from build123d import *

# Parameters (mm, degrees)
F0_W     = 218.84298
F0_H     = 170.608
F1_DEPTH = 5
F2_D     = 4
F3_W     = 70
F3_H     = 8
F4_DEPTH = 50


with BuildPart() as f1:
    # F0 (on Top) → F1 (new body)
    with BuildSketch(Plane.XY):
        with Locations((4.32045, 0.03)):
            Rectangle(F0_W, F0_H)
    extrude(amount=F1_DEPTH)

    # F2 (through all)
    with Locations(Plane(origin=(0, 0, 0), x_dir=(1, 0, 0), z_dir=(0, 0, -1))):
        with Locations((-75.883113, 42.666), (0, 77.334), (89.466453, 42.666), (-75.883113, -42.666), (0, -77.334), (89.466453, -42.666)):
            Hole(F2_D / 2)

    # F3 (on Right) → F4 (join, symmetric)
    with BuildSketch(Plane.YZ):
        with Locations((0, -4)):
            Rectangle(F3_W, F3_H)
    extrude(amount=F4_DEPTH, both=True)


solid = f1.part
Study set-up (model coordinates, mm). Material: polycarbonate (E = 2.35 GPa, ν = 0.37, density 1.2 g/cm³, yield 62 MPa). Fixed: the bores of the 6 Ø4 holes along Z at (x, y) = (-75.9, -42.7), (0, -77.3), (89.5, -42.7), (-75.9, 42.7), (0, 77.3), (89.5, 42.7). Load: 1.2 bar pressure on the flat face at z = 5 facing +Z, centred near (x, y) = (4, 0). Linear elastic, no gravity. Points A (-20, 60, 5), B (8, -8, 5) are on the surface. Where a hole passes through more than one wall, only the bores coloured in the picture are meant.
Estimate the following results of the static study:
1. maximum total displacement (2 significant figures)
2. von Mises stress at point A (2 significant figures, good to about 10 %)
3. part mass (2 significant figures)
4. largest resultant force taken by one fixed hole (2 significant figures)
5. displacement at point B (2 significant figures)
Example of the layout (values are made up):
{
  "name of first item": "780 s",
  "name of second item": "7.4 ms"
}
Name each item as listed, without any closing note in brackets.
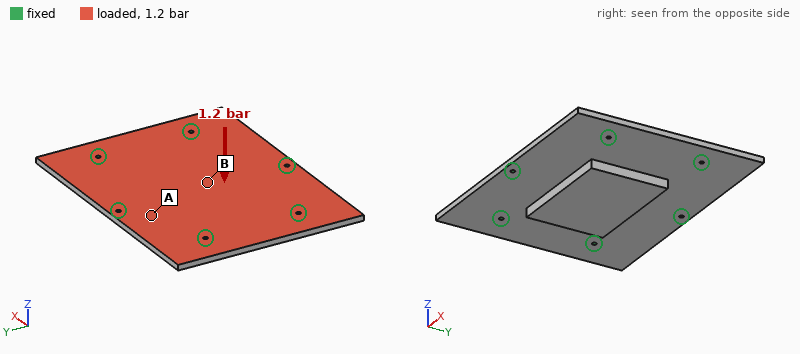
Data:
{
  "maximum total displacement": "2.2 mm",
  "von Mises stress at point A": "11 MPa",
  "part mass": "290 g",
  "largest resultant force taken by one fixed hole": "830 N",
  "displacement at point B": "2.0 mm"
}
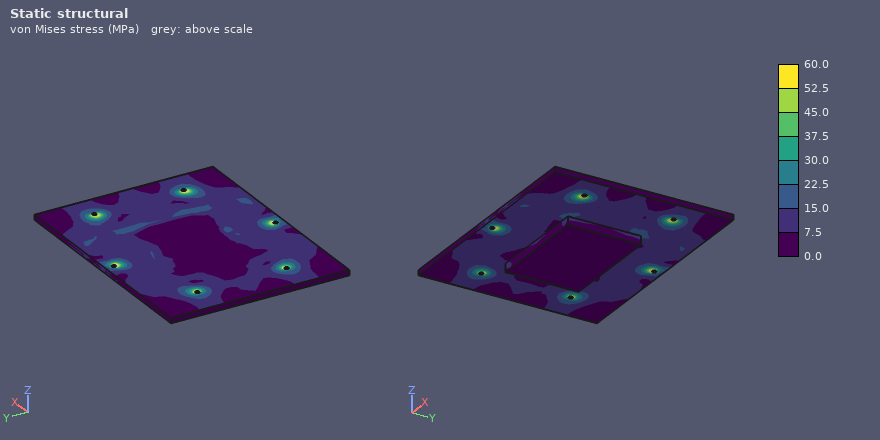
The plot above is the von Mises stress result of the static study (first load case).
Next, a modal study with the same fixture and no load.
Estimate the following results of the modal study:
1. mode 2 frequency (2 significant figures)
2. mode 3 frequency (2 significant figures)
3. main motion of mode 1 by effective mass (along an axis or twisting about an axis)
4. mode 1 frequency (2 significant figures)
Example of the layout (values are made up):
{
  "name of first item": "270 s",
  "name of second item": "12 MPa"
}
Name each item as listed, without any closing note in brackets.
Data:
{
  "mode 2 frequency": "570 Hz",
  "mode 3 frequency": "570 Hz",
  "main motion of mode 1 by effective mass": "along Z",
  "mode 1 frequency": "390 Hz"
}
